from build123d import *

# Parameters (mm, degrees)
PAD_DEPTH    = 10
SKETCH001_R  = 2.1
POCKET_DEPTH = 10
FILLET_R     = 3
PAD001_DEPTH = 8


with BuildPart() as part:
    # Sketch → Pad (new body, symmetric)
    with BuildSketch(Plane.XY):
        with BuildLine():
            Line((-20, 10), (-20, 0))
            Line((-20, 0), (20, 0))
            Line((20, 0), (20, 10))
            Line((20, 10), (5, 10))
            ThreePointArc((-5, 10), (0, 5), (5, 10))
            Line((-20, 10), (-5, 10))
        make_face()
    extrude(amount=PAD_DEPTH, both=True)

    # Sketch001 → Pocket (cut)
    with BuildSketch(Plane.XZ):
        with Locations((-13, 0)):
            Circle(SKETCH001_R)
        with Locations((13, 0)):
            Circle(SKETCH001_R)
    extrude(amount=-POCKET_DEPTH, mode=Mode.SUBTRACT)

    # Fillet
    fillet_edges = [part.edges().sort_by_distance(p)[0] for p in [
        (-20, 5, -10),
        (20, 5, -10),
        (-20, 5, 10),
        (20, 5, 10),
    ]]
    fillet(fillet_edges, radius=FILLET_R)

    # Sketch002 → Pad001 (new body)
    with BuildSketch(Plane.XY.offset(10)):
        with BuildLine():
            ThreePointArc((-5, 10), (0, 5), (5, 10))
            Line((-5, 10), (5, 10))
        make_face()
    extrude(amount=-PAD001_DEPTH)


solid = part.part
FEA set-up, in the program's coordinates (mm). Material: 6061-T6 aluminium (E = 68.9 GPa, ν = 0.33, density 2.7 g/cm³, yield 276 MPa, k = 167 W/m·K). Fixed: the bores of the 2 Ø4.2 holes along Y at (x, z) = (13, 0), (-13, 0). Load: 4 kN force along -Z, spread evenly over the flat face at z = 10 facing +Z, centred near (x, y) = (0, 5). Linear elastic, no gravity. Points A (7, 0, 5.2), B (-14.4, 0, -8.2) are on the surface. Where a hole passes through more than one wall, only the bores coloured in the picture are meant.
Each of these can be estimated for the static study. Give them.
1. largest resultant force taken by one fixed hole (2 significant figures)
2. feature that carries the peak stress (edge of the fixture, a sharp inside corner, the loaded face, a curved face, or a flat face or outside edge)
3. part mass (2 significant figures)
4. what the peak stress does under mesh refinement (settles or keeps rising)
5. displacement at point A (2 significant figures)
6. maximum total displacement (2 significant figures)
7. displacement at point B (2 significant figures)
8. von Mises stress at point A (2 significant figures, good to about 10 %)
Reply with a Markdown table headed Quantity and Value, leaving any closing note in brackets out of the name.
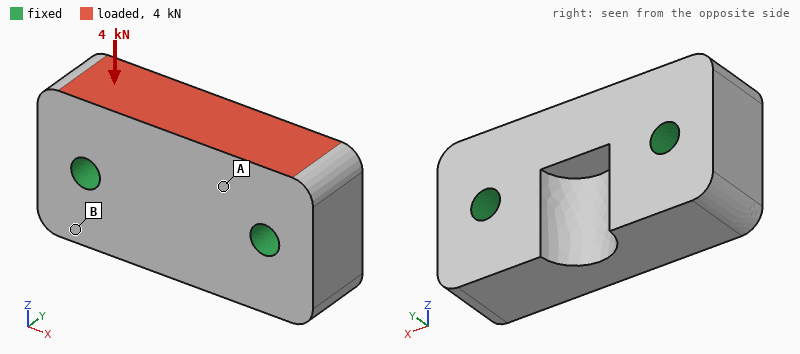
| Quantity | Value |
|---|---|
| largest resultant force taken by one fixed hole | 2.1 kN |
| feature that carries the peak stress | edge of the fixture |
| part mass | 19 g |
| what the peak stress does under mesh refinement | keeps rising |
| displacement at point A | 2.5 µm |
| maximum total displacement | 4.9 µm |
| displacement at point B | 0.78 µm |
| von Mises stress at point A | 12 MPa |
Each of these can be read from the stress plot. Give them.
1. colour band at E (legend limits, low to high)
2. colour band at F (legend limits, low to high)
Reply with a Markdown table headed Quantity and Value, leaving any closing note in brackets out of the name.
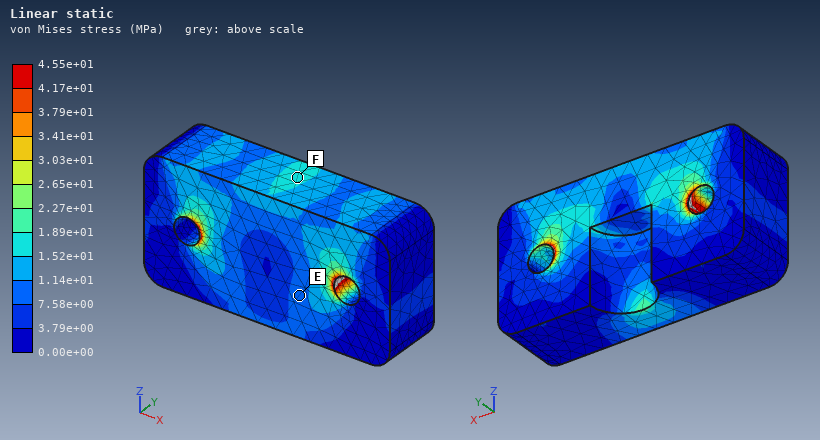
| Quantity | Value |
|---|---|
| colour band at E | 7.58e+00 to 1.14e+01 MPa |
| colour band at F | 1.52e+01 to 1.89e+01 MPa |
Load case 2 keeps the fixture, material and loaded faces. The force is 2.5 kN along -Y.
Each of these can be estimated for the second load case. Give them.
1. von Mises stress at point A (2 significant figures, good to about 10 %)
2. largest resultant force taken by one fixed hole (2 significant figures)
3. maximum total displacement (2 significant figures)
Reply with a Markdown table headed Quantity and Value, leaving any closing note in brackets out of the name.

| Quantity | Value |
|---|---|
| von Mises stress at point A | 21 MPa |
| largest resultant force taken by one fixed hole | 1.3 kN |
| maximum total displacement | 15 µm |
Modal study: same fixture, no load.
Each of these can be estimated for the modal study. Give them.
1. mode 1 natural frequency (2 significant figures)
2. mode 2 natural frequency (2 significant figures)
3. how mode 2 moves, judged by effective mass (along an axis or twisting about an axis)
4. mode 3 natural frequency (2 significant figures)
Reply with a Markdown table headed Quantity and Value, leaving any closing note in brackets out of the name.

| Quantity | Value |
|---|---|
| mode 1 natural frequency | 38 kHz |
| mode 2 natural frequency | 40 kHz |
| how mode 2 moves, judged by effective mass | along Y |
| mode 3 natural frequency | 46 kHz |
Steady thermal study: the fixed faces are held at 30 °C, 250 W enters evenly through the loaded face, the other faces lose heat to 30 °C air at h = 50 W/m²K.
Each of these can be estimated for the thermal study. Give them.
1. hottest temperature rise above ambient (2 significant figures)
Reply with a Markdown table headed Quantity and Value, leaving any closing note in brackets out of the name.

| Quantity | Value |
|---|---|
| hottest temperature rise above ambient | 57 K |
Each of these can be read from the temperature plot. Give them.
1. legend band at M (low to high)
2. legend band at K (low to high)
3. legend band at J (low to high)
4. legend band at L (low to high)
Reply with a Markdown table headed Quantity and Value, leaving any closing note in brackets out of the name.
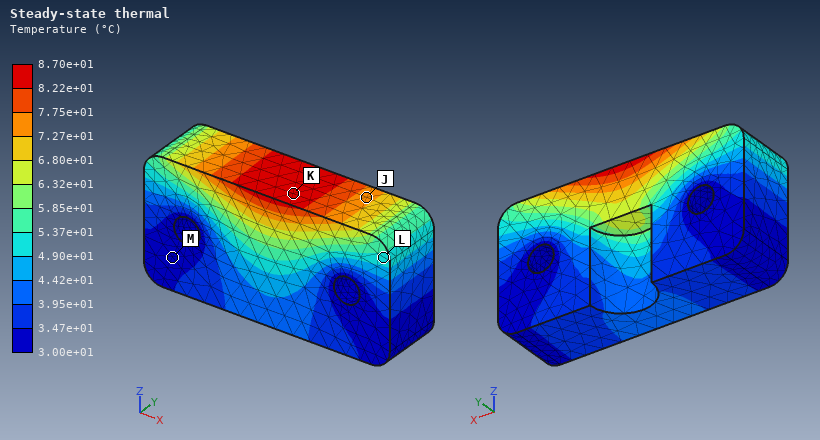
| Quantity | Value |
|---|---|
| legend band at M | 3.00e+01 to 3.47e+01 °C |
| legend band at K | 8.22e+01 to 8.70e+01 °C |
| legend band at J | 7.27e+01 to 7.75e+01 °C |
| legend band at L | 4.90e+01 to 5.37e+01 °C |
